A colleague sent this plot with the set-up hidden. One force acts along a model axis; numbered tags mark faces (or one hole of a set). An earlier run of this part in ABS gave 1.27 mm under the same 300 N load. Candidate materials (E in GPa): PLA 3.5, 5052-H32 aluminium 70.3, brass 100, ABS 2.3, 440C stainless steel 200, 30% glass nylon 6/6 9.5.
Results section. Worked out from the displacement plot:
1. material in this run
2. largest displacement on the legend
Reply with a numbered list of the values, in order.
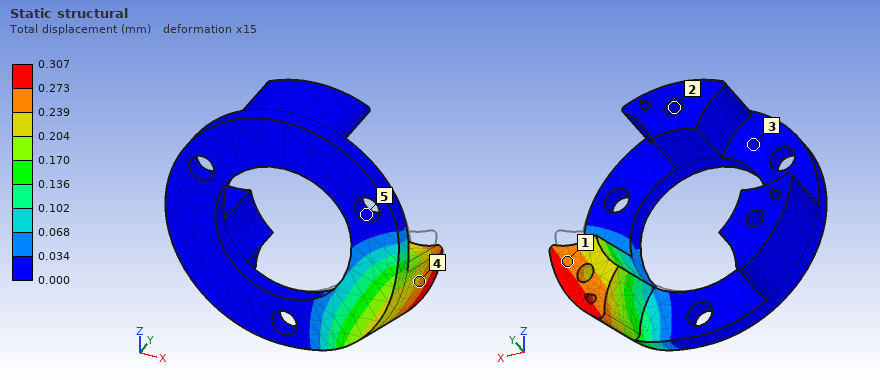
1. 30% glass nylon 6/6
2. 0.307 mm
